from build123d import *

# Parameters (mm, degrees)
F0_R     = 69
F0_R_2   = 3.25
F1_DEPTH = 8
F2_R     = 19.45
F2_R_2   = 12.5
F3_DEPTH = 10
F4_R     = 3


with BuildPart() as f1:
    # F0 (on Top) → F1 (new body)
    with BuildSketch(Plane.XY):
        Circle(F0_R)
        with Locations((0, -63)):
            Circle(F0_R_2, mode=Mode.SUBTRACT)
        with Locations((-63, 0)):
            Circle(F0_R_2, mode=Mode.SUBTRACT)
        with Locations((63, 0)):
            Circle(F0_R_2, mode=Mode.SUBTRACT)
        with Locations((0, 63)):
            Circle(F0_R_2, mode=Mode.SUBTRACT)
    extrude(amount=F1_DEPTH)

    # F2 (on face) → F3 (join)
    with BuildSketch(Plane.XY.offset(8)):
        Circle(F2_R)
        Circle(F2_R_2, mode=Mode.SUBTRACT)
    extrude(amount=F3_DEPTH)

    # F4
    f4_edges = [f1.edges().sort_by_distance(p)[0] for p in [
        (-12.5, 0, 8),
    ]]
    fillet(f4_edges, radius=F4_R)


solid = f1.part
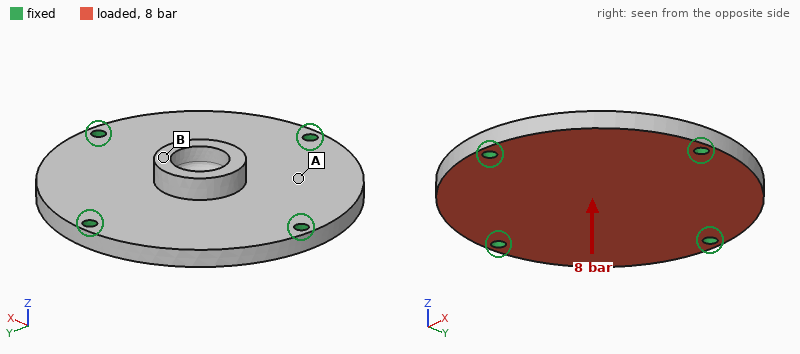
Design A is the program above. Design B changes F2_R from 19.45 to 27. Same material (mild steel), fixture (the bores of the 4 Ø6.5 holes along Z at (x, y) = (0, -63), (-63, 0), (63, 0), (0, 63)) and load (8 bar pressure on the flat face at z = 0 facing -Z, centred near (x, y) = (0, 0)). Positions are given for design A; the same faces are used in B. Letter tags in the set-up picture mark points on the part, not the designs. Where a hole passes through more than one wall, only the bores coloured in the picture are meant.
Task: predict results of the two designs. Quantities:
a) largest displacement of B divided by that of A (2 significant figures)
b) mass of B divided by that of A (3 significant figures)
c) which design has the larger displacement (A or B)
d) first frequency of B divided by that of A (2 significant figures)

0.81
1.09
A
1.0
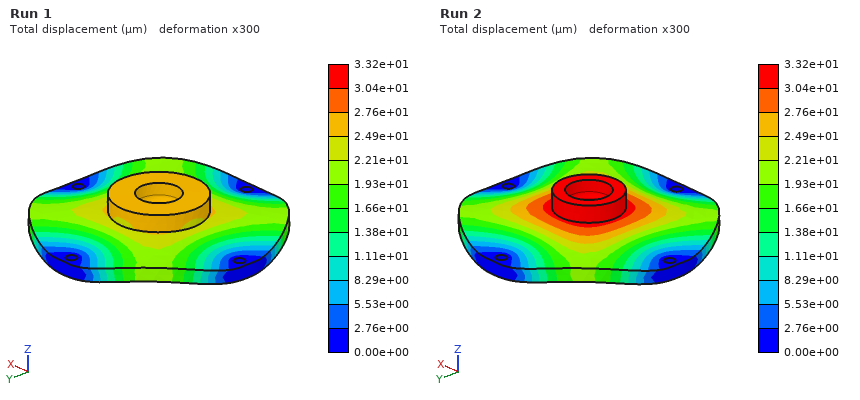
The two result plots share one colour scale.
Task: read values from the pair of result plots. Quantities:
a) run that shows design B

Run 1
